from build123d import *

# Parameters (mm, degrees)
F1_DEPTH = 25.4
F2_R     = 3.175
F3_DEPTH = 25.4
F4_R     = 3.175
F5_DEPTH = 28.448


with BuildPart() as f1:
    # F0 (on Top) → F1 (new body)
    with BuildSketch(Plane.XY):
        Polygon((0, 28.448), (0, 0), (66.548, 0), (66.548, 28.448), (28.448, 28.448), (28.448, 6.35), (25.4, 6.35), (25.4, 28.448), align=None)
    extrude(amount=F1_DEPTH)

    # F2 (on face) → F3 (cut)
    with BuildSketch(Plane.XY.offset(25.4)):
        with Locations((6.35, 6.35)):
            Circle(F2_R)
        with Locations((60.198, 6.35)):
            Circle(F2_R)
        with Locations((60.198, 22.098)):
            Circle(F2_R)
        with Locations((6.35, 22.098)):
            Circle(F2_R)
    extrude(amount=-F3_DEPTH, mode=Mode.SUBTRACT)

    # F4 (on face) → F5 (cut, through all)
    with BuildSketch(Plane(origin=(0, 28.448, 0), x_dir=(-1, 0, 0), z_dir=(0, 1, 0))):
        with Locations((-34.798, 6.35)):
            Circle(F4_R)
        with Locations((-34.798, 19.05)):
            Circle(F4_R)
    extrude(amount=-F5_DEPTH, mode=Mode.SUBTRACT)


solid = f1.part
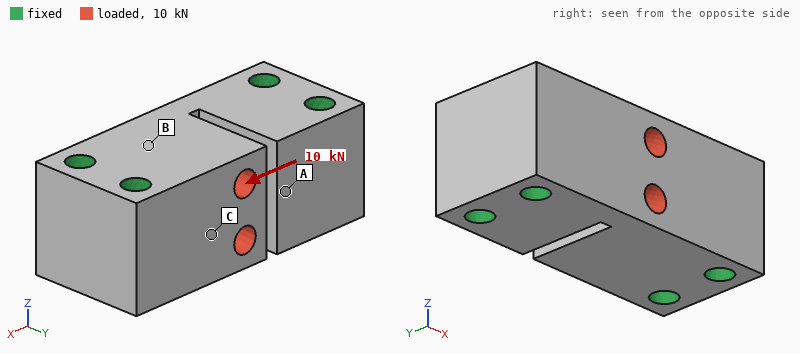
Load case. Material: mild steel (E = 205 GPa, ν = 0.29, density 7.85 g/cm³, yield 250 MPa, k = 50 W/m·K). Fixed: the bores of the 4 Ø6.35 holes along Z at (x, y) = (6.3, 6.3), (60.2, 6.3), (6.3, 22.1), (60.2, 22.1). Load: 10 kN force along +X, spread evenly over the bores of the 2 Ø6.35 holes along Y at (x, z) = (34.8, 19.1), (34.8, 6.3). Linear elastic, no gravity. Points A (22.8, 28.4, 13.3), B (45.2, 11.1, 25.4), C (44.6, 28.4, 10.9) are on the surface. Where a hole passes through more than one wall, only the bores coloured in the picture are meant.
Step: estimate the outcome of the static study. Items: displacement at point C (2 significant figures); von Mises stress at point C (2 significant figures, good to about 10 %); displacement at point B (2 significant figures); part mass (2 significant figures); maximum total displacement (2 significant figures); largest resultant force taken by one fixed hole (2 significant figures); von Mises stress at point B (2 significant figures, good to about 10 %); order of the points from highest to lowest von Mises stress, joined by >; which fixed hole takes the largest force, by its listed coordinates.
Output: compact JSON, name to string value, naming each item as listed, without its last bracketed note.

{"displacement at point C": "1.1 µm", "von Mises stress at point C": "16 MPa", "displacement at point B": "0.79 µm", "part mass": "320 g", "maximum total displacement": "2.5 µm", "largest resultant force taken by one fixed hole": "4.8 kN", "von Mises stress at point B": "11 MPa", "order of the points from highest to lowest von Mises stress, joined by >": "C > B > A", "which fixed hole takes the largest force, by its listed coordinates": "(60.2, 22.1)"}
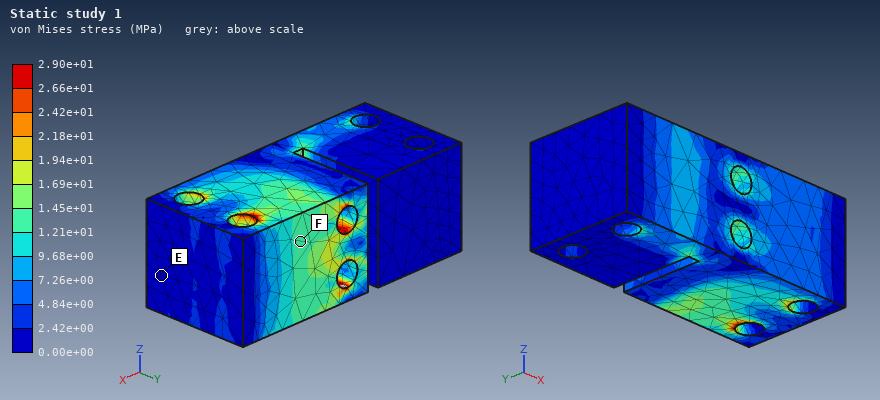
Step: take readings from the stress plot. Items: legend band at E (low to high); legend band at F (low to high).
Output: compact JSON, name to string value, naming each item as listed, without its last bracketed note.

{"legend band at E": "0.00e+00 to 2.42e+00 MPa", "legend band at F": "1.21e+01 to 1.45e+01 MPa"}
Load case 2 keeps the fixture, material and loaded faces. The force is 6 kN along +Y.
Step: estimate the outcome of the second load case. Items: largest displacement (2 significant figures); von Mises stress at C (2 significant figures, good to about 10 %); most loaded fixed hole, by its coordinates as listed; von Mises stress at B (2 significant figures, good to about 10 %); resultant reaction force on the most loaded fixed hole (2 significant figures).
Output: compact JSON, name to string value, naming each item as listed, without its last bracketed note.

{"largest displacement": "4.4 µm", "von Mises stress at C": "8.6 MPa", "most loaded fixed hole, by its coordinates as listed": "(60.2, 22.1)", "von Mises stress at B": "17 MPa", "resultant reaction force on the most loaded fixed hole": "4.8 kN"}
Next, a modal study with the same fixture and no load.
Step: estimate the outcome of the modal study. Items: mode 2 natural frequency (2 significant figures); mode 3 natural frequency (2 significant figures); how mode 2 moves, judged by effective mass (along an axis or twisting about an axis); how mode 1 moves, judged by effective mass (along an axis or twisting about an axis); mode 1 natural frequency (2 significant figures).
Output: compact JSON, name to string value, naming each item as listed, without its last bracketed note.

{"mode 2 natural frequency": "23 kHz", "mode 3 natural frequency": "29 kHz", "how mode 2 moves, judged by effective mass": "along Y", "how mode 1 moves, judged by effective mass": "along Z", "mode 1 natural frequency": "22 kHz"}
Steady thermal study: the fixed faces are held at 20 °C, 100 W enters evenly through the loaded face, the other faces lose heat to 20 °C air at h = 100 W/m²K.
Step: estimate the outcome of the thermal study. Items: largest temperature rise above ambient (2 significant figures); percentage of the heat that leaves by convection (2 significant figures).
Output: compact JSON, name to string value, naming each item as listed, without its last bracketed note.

{"largest temperature rise above ambient": "56 K", "percentage of the heat that leaves by convection": "13 %"}
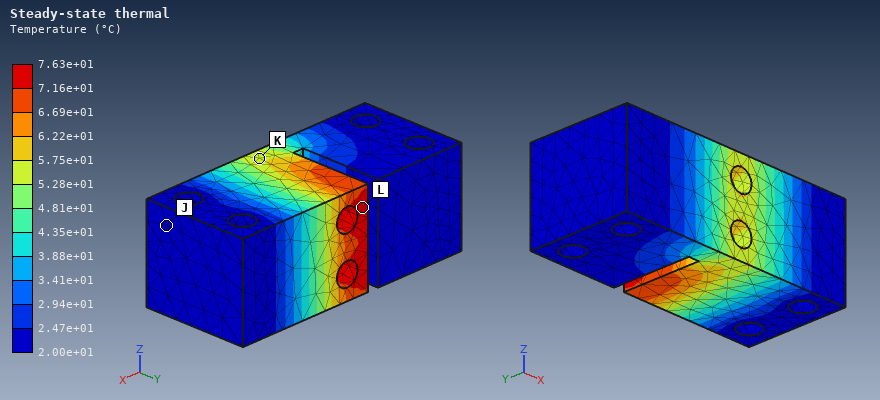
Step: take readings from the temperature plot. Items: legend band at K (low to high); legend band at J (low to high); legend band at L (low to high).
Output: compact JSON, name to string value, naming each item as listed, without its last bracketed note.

{"legend band at K": "5.28e+01 to 5.75e+01 °C", "legend band at J": "2.00e+01 to 2.47e+01 °C", "legend band at L": "7.16e+01 to 7.63e+01 °C"}
